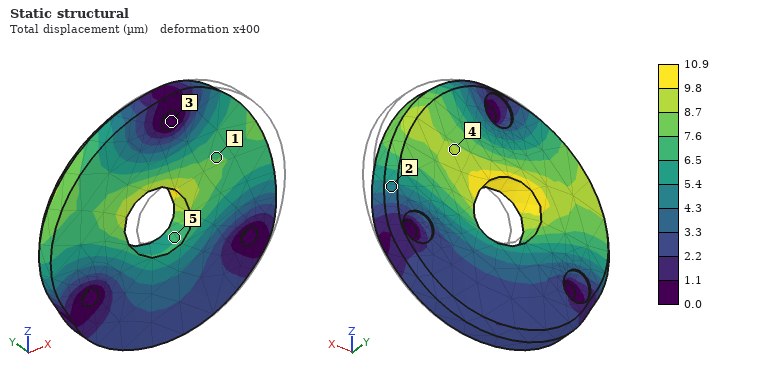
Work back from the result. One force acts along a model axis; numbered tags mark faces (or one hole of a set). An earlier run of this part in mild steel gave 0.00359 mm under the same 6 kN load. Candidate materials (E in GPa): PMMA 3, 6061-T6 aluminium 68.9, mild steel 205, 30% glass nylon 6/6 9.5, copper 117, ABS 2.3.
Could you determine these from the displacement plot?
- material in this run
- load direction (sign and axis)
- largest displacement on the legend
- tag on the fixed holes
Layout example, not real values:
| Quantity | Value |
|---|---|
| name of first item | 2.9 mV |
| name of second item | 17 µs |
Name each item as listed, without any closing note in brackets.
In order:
| Quantity | Value |
|---|---|
| material in this run | 6061-T6 aluminium |
| load direction | -X |
| largest displacement on the legend | 10.9 µm |
| tag on the fixed holes | 3 |
